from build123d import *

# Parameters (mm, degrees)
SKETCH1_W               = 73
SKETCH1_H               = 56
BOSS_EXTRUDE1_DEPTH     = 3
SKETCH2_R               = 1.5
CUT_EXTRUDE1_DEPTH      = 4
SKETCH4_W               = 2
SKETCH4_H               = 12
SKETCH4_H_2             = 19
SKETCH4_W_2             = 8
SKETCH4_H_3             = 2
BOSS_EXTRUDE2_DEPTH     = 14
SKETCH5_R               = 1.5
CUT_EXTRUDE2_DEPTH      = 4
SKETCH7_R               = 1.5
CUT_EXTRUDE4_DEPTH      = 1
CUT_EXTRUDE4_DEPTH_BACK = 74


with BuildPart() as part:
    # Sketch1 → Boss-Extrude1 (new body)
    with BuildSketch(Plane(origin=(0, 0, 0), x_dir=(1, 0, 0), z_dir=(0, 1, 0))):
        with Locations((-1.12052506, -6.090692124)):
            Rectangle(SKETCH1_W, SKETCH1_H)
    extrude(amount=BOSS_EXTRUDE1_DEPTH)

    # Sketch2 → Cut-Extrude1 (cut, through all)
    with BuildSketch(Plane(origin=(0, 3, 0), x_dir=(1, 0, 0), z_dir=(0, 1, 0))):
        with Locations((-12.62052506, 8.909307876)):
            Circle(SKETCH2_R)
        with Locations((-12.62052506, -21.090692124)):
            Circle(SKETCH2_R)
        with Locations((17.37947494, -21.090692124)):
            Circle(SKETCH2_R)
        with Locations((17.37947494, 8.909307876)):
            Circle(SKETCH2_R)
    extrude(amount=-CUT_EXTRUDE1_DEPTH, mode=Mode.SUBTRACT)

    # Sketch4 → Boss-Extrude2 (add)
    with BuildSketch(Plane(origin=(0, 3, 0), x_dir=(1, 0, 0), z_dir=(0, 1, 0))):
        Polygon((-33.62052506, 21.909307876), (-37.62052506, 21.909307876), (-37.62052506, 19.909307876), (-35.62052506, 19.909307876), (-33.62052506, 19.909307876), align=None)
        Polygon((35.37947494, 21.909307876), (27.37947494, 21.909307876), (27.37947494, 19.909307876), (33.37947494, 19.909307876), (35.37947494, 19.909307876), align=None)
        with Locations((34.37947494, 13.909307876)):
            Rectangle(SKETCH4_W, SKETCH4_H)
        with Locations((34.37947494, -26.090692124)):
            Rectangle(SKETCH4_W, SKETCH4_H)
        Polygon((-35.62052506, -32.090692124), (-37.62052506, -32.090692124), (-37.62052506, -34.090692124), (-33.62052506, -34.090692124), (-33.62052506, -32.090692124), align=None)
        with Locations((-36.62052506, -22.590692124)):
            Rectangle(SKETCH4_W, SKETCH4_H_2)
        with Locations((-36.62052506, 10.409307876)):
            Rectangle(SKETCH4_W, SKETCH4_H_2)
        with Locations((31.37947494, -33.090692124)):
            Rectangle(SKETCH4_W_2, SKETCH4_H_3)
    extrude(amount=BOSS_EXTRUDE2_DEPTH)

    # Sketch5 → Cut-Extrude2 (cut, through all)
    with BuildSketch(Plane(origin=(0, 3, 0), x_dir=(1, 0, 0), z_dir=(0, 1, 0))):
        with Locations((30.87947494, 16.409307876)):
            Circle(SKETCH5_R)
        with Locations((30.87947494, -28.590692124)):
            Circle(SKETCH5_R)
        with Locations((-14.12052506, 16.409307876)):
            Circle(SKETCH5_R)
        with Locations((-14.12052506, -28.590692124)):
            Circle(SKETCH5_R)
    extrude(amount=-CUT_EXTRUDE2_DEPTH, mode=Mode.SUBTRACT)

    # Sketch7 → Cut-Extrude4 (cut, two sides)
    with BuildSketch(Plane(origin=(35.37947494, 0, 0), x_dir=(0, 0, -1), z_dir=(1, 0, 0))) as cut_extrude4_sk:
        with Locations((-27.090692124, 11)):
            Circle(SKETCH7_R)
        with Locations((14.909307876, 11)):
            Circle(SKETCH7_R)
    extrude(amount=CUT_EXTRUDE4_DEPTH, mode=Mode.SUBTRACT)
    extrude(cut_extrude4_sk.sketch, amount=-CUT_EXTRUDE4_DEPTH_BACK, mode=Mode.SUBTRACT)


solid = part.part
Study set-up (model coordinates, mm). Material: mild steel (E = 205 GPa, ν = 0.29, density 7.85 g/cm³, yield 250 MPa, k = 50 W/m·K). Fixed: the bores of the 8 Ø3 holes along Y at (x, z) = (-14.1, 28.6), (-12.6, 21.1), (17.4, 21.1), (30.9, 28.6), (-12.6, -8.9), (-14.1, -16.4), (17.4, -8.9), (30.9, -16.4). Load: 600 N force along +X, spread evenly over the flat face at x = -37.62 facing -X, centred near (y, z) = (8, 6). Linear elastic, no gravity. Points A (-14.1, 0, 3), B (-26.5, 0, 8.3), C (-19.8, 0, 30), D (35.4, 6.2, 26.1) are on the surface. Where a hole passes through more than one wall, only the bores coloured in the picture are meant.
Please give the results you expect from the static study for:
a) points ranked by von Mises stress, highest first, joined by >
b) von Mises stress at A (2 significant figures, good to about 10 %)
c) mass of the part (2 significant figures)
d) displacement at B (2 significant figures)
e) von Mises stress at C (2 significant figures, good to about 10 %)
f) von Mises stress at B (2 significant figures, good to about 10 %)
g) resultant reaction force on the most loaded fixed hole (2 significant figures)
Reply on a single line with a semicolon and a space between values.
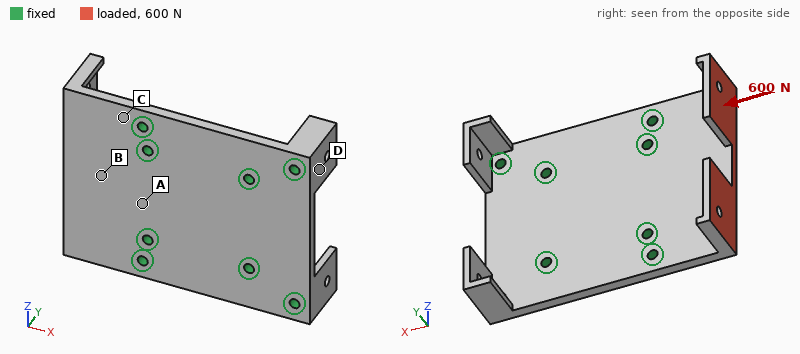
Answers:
C > B > A > D; 25 MPa; 110 g; 16 µm; 48 MPa; 35 MPa; 140 N
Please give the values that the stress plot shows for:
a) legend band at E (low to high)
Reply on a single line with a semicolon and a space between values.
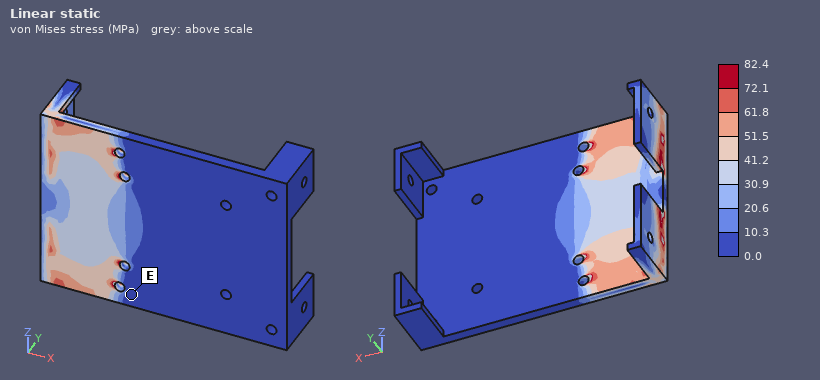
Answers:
0.0 to 10.3 MPa
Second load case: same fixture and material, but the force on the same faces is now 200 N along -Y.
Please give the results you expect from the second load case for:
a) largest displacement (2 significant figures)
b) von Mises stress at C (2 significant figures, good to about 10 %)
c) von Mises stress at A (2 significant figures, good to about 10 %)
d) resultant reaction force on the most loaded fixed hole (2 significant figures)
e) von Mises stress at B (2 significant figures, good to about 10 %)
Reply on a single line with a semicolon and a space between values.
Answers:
53 µm; 49 MPa; 26 MPa; 59 N; 23 MPa
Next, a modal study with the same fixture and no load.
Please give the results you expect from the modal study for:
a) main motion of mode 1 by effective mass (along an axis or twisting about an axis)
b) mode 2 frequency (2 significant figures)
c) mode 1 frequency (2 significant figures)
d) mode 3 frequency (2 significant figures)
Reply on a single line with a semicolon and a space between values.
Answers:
along Y; 3500 Hz; 2600 Hz; 5600 Hz
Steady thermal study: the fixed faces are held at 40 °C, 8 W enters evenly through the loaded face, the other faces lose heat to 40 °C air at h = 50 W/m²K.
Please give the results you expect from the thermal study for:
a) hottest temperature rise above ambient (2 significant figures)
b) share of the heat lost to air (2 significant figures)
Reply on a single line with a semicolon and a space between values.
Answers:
27 K; 32 %
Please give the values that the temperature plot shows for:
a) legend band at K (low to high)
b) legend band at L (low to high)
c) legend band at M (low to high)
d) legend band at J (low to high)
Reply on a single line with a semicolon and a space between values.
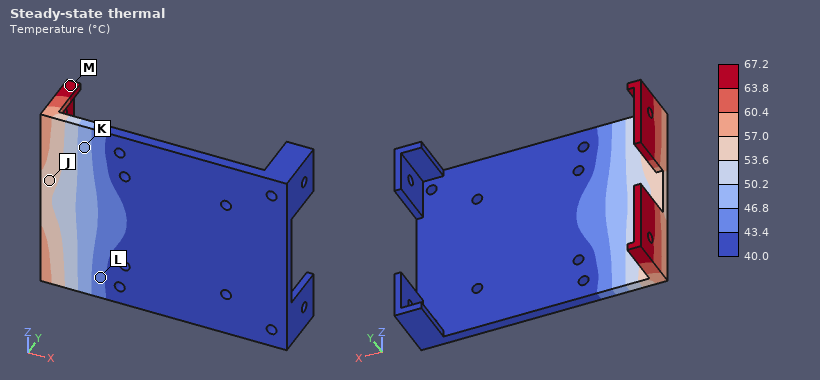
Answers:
46.8 to 50.2 °C; 43.4 to 46.8 °C; 63.8 to 67.2 °C; 53.6 to 57.0 °C
